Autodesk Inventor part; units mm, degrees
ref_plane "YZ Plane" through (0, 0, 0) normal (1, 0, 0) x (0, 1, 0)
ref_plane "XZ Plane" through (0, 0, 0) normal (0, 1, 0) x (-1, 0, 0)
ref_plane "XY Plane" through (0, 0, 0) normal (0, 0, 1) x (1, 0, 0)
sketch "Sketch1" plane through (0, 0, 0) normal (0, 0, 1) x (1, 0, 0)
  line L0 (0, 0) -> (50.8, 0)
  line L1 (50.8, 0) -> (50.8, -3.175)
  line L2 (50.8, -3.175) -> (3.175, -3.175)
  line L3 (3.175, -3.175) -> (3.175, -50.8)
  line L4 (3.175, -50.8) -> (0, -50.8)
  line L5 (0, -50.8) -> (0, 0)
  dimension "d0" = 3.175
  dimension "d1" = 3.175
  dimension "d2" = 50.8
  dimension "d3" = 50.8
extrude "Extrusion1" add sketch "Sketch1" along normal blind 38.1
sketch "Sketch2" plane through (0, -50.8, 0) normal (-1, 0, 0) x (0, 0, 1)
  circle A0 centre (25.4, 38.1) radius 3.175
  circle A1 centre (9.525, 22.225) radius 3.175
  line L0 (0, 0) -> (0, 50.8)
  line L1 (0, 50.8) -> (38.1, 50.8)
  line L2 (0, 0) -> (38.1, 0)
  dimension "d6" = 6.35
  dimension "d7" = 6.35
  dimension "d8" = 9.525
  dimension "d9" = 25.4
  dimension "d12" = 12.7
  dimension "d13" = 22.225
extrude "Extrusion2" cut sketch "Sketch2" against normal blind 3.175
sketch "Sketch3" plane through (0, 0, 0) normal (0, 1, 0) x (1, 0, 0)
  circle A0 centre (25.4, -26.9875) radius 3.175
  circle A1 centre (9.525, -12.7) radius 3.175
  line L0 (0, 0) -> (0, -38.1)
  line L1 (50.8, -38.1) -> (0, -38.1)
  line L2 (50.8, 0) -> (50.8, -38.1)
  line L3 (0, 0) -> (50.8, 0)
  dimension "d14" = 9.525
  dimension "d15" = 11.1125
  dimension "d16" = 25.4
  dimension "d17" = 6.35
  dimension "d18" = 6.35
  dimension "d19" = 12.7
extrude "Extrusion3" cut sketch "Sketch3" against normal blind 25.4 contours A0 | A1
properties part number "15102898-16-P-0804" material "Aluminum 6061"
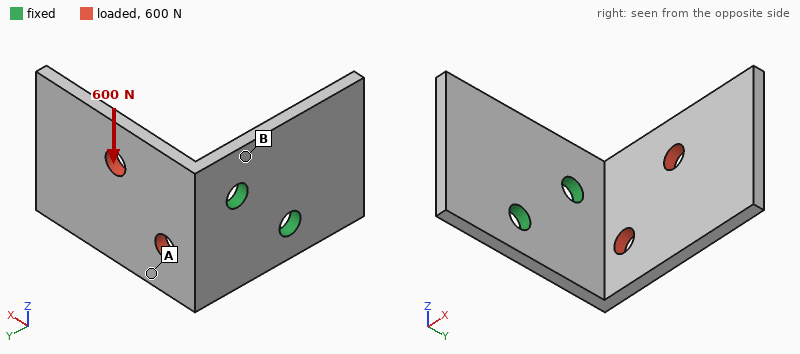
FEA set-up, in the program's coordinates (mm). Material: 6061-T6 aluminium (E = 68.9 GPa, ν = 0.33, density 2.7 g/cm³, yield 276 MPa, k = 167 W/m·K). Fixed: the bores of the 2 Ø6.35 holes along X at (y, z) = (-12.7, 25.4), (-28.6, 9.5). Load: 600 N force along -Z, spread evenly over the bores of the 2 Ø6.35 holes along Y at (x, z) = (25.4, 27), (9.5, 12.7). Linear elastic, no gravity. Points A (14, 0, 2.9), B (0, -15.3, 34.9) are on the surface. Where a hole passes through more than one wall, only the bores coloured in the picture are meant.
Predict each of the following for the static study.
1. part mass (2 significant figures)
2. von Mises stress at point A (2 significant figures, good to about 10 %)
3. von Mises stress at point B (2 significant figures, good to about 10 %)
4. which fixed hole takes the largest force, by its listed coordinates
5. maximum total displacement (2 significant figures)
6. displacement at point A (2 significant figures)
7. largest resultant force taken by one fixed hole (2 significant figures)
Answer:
31 g
22 MPa
59 MPa
(-12.7, 25.4)
0.40 mm
0.18 mm
700 N
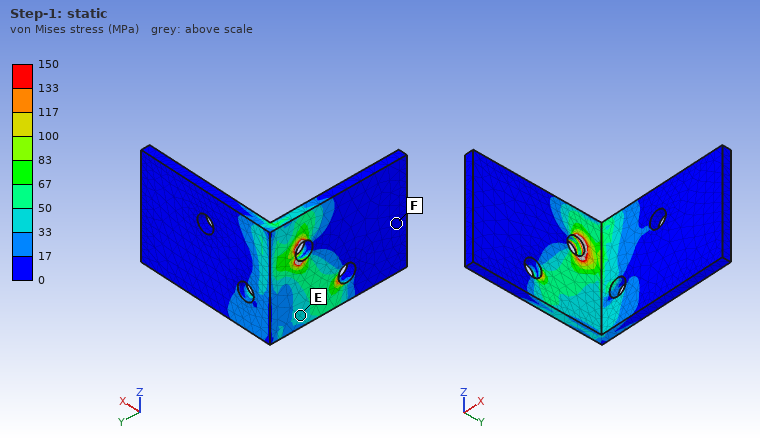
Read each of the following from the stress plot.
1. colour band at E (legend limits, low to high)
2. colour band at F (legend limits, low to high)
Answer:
33 to 50 MPa
0 to 17 MPa
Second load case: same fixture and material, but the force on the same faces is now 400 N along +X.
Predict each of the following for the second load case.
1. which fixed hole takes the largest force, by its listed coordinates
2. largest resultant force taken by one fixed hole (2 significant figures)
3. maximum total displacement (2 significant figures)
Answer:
(-12.7, 25.4)
400 N
0.21 mm
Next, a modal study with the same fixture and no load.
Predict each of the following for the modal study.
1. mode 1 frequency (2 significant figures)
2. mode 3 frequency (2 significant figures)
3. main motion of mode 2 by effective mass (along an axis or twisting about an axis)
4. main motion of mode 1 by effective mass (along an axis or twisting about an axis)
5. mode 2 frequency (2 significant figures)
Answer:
790 Hz
2900 Hz
along Z
along Y
1500 Hz
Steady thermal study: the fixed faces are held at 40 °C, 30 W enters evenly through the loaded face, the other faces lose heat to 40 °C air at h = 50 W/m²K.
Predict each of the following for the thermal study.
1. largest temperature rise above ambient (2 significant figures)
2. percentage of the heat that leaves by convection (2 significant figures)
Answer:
39 K
22 %
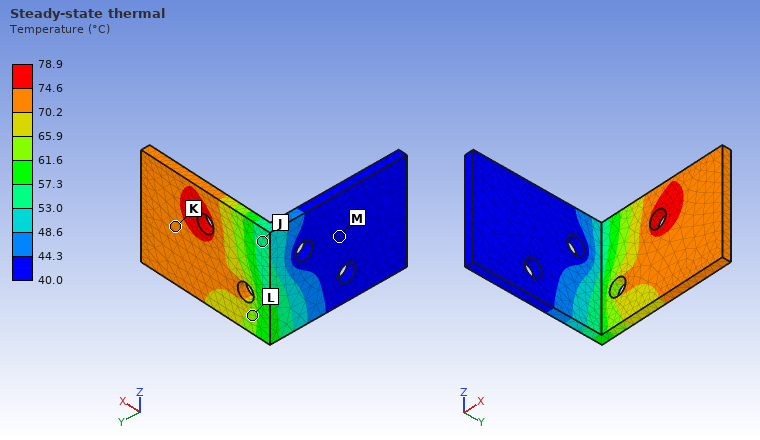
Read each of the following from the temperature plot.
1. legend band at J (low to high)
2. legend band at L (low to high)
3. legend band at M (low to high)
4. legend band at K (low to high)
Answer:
53.0 to 57.3 °C
61.6 to 65.9 °C
40.0 to 44.3 °C
70.2 to 74.6 °C
